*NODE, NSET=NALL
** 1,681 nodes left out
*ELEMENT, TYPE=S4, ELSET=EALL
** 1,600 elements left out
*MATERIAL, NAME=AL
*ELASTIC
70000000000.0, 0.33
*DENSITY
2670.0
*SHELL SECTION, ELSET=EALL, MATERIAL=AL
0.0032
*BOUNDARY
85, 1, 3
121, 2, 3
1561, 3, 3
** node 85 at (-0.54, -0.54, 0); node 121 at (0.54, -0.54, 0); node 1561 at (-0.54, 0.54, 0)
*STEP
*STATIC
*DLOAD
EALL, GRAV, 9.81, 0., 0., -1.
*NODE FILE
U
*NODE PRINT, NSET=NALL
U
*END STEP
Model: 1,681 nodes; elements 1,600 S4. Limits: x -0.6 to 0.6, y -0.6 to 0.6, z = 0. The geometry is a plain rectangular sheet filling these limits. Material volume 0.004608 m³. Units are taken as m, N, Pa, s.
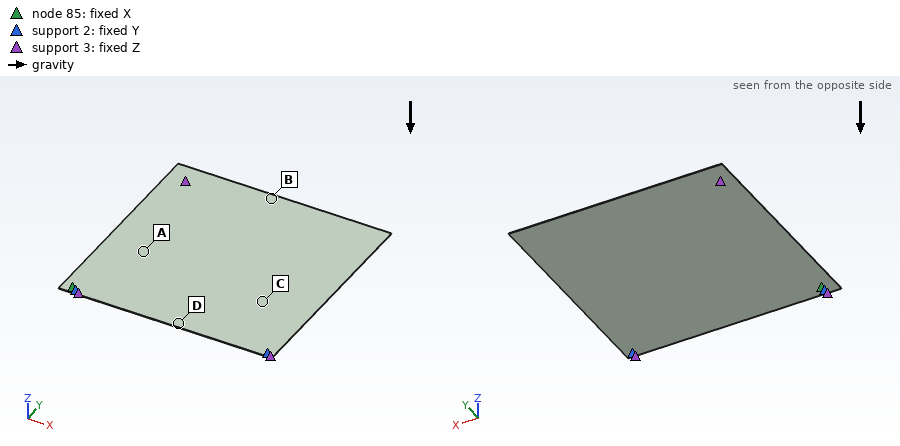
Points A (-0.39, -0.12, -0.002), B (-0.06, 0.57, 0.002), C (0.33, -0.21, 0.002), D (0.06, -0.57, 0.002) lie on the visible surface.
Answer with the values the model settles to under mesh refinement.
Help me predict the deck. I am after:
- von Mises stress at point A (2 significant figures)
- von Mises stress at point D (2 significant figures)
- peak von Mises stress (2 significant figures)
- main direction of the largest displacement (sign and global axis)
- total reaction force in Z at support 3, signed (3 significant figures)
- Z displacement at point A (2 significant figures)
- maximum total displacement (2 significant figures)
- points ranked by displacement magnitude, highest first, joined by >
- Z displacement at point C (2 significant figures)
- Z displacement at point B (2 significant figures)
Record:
1.3e+07 Pa
1.6e+07 Pa
1.7e+07 Pa
-Z
121 N
-0.015 m
0.11 m
B > C > A > D
-0.034 m
-0.054 m
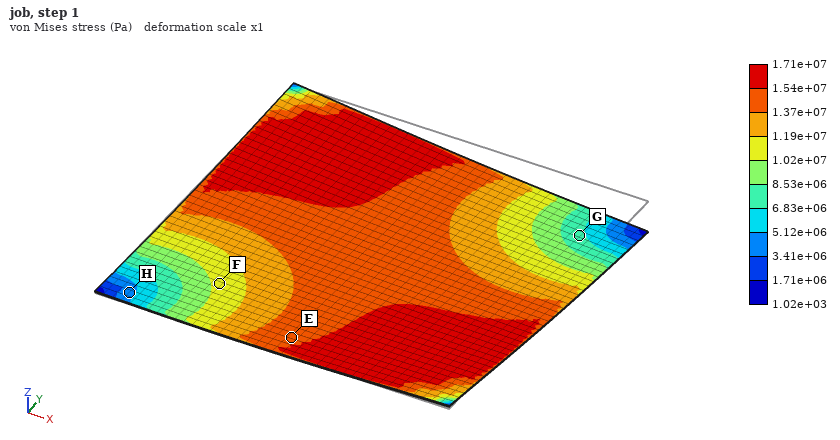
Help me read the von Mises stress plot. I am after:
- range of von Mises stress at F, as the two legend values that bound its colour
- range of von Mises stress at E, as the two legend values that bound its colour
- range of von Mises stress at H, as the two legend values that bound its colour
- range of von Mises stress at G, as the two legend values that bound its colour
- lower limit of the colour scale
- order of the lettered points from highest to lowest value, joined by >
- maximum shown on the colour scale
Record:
1.02e+07 to 1.19e+07 Pa
1.37e+07 to 1.54e+07 Pa
3.41e+06 to 5.12e+06 Pa
6.83e+06 to 8.53e+06 Pa
1.02e+03 Pa
E > F > G > H
1.71e+07 Pa
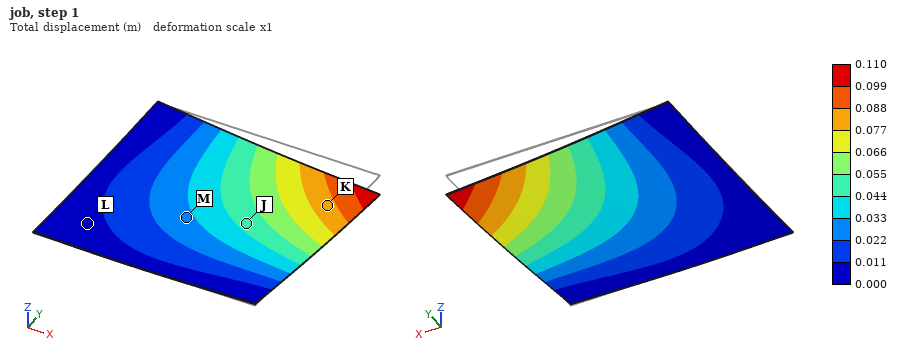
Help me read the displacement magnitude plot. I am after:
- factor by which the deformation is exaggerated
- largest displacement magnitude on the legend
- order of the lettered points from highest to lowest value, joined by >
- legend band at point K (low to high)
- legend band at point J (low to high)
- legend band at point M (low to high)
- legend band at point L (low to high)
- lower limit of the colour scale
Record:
1
0.110 m
K > J > M > L
0.077 to 0.088 m
0.044 to 0.055 m
0.022 to 0.033 m
0.000 to 0.011 m
0.000 m
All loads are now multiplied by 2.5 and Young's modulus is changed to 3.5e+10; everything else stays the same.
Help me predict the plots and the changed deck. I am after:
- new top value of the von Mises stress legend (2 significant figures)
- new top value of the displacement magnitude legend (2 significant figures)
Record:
4.3e+07 Pa
0.55 m
